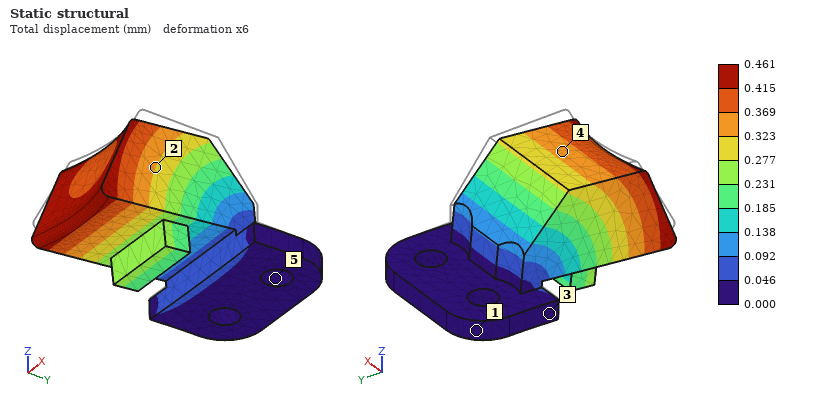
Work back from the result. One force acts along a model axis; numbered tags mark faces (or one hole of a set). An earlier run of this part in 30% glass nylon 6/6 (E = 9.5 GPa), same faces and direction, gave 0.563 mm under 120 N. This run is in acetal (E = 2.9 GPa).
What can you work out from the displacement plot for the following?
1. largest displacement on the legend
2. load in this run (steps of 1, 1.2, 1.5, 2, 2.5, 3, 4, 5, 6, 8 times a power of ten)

0.461 mm
30 N
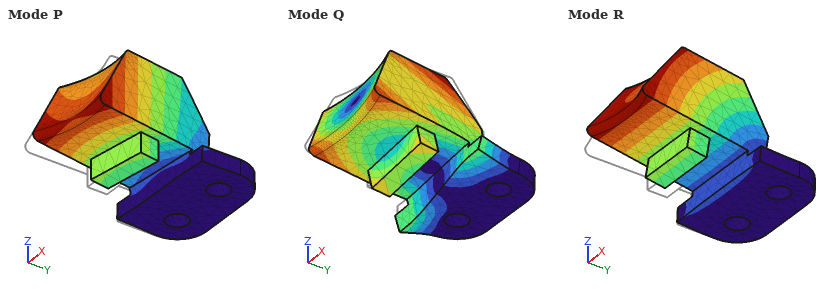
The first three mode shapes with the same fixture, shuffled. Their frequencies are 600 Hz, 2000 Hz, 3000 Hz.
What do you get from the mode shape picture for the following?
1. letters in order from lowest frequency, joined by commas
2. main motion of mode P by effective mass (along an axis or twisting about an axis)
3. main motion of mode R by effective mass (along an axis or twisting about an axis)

R, P, Q
along X
along Z
